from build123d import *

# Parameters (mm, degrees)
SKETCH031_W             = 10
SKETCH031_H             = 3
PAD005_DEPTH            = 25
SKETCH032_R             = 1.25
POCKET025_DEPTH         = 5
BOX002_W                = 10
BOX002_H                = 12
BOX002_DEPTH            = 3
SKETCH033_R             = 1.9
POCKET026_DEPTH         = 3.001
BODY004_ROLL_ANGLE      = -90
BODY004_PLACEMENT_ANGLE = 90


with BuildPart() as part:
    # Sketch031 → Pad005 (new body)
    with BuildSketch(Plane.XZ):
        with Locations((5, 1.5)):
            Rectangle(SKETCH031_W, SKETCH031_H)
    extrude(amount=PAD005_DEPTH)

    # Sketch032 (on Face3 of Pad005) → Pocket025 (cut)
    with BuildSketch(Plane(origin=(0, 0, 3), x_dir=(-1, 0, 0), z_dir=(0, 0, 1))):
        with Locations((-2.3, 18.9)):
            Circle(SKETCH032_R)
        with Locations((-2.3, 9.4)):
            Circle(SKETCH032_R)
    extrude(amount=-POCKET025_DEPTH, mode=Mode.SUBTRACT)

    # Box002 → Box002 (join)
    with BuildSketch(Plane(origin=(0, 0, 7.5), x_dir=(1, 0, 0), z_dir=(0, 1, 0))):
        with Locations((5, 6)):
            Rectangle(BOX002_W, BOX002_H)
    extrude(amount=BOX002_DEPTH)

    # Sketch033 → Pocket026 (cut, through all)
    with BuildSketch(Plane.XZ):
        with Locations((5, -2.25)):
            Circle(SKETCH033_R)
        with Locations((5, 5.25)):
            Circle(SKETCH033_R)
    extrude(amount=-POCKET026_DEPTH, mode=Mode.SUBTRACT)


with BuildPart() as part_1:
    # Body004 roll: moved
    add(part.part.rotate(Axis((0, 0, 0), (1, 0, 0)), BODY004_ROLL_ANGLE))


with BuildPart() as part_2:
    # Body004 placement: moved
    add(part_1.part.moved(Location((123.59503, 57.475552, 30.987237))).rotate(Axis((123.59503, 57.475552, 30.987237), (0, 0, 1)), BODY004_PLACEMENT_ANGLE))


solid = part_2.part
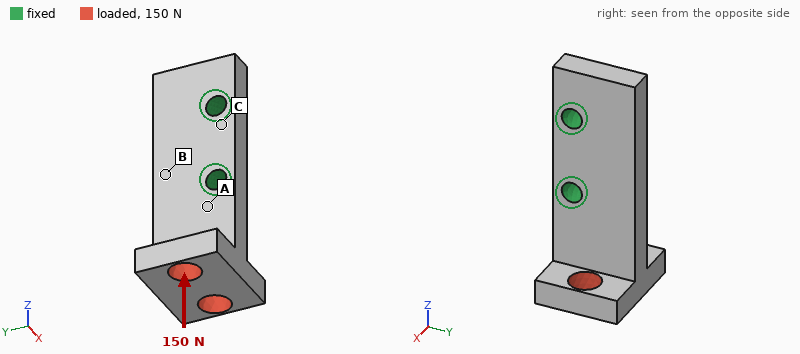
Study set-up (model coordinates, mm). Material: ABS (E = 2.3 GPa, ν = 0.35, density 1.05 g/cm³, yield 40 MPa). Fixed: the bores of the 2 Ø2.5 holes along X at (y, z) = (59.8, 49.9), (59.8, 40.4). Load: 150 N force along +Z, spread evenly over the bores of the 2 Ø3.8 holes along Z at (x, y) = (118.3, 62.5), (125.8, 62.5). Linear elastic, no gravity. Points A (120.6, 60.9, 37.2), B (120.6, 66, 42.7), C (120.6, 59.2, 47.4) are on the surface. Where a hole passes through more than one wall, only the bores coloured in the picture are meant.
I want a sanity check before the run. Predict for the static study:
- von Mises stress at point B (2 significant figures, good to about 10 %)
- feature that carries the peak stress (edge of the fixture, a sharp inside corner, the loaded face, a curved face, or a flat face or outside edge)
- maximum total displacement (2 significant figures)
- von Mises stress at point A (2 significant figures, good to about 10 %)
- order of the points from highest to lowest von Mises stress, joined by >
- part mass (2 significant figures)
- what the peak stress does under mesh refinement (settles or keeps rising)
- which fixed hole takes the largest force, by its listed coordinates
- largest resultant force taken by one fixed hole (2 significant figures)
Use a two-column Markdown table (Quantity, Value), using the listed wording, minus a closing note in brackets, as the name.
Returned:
| Quantity | Value |
|---|---|
| von Mises stress at point B | 3.9 MPa |
| feature that carries the peak stress | a sharp inside corner |
| maximum total displacement | 0.13 mm |
| von Mises stress at point A | 6.9 MPa |
| order of the points from highest to lowest von Mises stress, joined by > | A > B > C |
| part mass | 1.1 g |
| what the peak stress does under mesh refinement | keeps rising |
| which fixed hole takes the largest force, by its listed coordinates | (59.8, 40.4) |
| largest resultant force taken by one fixed hole | 120 N |
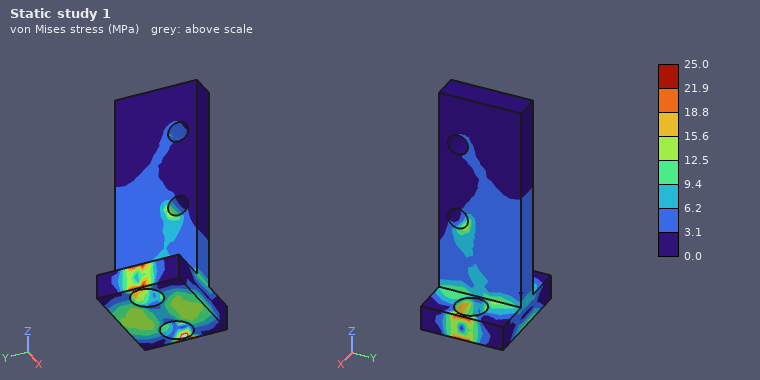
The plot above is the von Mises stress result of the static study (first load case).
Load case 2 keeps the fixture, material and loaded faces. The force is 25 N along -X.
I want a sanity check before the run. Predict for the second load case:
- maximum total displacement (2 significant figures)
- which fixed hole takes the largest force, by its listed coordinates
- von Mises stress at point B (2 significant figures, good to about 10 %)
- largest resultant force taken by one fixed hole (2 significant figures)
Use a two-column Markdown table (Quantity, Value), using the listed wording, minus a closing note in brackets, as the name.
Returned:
| Quantity | Value |
|---|---|
| maximum total displacement | 0.35 mm |
| which fixed hole takes the largest force, by its listed coordinates | (59.8, 40.4) |
| von Mises stress at point B | 5.5 MPa |
| largest resultant force taken by one fixed hole | 33 N |
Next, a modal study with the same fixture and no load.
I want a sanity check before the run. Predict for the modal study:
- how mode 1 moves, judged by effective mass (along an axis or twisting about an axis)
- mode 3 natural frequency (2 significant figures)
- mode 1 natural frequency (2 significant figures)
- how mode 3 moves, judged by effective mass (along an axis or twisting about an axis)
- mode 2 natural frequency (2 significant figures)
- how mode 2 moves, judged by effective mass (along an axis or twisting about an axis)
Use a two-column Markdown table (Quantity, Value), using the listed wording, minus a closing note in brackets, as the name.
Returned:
| Quantity | Value |
|---|---|
| how mode 1 moves, judged by effective mass | along X |
| mode 3 natural frequency | 5600 Hz |
| mode 1 natural frequency | 2600 Hz |
| how mode 3 moves, judged by effective mass | along Y |
| mode 2 natural frequency | 4800 Hz |
| how mode 2 moves, judged by effective mass | twisting about Z |
